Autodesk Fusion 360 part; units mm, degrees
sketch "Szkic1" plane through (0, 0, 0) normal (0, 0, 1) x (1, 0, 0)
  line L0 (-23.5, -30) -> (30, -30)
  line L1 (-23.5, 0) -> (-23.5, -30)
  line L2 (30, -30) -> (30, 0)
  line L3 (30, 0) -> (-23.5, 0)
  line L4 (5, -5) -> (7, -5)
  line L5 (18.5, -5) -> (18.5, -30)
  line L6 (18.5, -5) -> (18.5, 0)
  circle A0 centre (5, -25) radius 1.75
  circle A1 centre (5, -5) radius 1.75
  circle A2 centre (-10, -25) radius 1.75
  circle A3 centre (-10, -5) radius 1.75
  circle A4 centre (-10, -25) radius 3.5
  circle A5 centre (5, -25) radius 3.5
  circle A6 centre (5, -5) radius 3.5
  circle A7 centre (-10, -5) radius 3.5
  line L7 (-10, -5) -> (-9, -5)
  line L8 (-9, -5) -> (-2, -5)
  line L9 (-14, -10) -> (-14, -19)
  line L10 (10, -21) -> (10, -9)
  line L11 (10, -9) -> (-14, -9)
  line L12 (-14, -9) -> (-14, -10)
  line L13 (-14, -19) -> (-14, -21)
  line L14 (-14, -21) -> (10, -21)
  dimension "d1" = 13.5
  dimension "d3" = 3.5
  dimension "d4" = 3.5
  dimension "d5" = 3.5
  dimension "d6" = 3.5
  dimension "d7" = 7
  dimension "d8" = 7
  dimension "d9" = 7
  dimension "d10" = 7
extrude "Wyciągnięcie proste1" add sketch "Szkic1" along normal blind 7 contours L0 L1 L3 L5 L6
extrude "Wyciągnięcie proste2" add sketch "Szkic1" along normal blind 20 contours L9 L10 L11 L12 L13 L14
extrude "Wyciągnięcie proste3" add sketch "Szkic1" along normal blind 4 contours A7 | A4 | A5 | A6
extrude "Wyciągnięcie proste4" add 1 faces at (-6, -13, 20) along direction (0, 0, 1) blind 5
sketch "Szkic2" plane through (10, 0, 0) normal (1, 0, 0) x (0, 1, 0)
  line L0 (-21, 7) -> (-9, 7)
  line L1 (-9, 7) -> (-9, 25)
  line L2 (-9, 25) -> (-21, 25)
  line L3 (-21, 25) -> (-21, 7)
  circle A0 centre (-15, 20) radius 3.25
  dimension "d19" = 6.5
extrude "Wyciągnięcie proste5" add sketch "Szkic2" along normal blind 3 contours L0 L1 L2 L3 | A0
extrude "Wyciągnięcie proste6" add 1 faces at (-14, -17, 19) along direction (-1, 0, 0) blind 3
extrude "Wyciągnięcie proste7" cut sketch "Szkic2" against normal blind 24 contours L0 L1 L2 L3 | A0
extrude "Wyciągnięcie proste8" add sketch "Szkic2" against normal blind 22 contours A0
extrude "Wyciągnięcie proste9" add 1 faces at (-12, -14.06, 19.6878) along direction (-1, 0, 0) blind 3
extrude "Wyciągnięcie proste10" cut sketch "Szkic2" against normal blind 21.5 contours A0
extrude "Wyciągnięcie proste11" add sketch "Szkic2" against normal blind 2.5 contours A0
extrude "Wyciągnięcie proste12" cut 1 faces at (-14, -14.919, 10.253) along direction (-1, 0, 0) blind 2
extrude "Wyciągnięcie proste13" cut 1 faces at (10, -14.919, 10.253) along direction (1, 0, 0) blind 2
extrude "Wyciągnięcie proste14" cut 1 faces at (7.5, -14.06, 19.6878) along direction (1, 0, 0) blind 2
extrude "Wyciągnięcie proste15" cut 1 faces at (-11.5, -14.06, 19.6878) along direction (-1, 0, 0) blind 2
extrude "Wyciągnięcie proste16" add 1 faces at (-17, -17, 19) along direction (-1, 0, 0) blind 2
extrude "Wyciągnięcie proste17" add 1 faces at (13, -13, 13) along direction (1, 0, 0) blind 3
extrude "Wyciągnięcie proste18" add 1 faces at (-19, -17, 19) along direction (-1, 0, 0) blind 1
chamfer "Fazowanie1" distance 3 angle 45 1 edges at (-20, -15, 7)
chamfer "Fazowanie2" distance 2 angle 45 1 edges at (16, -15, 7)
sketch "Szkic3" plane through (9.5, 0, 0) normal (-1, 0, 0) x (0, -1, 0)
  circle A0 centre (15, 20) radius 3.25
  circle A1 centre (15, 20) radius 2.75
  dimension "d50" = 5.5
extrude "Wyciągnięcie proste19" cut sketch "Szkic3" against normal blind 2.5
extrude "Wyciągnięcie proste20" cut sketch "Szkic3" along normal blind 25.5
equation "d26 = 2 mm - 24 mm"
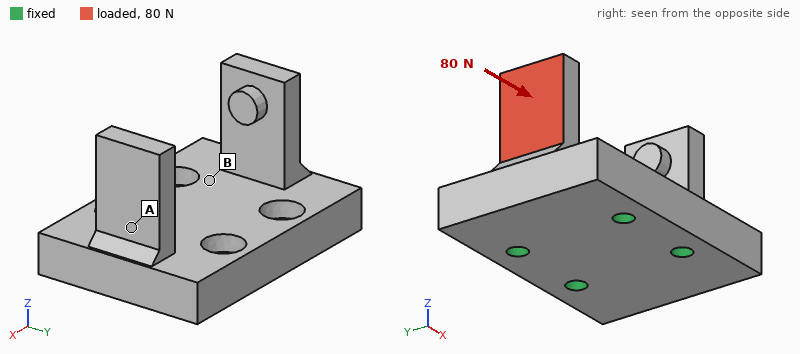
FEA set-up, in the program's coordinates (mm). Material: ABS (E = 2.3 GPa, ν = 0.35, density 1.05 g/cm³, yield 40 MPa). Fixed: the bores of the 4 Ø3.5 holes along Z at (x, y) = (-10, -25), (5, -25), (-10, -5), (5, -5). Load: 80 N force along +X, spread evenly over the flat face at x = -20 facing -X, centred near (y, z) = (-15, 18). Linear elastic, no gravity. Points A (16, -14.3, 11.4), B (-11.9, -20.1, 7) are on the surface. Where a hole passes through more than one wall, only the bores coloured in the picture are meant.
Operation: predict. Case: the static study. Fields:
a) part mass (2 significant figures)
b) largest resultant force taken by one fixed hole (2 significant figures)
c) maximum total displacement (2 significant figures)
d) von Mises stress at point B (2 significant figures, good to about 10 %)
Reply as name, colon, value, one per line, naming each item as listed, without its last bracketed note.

part mass: 11 g
largest resultant force taken by one fixed hole: 47 N
maximum total displacement: 0.61 mm
von Mises stress at point B: 5.9 MPa
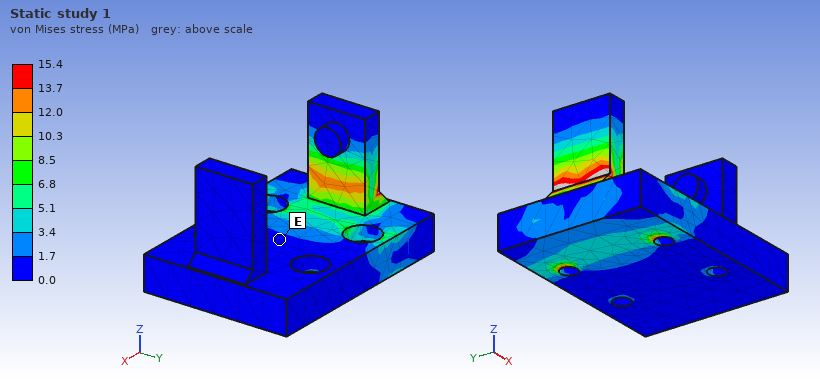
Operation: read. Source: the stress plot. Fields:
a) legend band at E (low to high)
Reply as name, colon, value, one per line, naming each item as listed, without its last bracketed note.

legend band at E: 0.0 to 1.7 MPa
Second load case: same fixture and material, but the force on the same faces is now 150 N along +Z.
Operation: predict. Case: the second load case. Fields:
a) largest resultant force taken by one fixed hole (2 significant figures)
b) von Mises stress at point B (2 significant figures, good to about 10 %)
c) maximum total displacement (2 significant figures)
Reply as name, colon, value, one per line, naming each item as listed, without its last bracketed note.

largest resultant force taken by one fixed hole: 110 N
von Mises stress at point B: 5.6 MPa
maximum total displacement: 0.40 mm
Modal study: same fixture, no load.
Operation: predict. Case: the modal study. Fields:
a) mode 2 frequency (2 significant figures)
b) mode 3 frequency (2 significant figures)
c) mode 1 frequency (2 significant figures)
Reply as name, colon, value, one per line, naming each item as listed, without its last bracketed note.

mode 2 frequency: 2400 Hz
mode 3 frequency: 4300 Hz
mode 1 frequency: 2200 Hz
